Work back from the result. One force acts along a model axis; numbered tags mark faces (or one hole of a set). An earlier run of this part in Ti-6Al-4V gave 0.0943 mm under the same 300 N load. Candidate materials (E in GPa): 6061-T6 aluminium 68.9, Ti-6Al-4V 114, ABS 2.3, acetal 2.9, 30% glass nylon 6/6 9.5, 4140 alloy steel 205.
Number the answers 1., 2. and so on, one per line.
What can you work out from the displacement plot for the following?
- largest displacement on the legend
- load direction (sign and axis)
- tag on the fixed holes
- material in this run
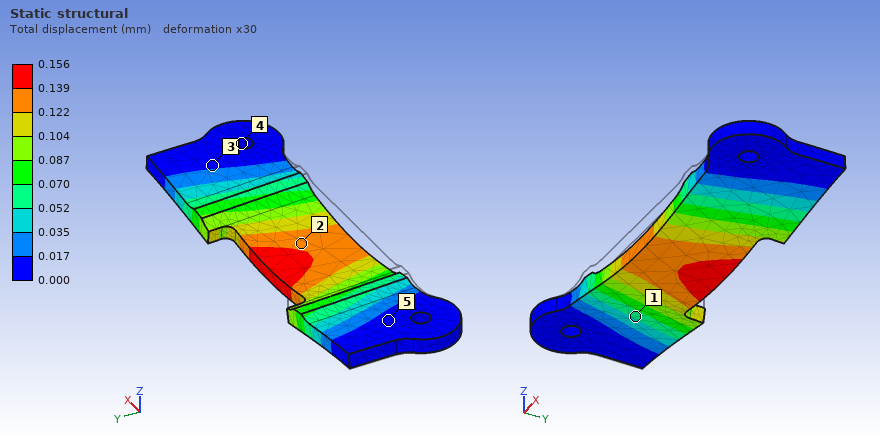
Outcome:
1. 0.156 mm
2. -Z
3. 4
4. 6061-T6 aluminium
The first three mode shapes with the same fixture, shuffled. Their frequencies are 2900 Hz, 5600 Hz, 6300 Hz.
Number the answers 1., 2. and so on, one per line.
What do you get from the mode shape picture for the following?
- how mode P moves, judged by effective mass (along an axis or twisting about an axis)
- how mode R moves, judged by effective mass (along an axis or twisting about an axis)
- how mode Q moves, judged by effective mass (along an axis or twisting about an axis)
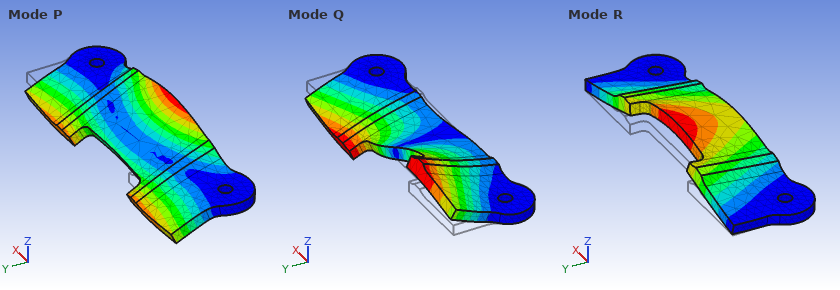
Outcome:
1. twisting about X
2. along Z
3. twisting about Y
